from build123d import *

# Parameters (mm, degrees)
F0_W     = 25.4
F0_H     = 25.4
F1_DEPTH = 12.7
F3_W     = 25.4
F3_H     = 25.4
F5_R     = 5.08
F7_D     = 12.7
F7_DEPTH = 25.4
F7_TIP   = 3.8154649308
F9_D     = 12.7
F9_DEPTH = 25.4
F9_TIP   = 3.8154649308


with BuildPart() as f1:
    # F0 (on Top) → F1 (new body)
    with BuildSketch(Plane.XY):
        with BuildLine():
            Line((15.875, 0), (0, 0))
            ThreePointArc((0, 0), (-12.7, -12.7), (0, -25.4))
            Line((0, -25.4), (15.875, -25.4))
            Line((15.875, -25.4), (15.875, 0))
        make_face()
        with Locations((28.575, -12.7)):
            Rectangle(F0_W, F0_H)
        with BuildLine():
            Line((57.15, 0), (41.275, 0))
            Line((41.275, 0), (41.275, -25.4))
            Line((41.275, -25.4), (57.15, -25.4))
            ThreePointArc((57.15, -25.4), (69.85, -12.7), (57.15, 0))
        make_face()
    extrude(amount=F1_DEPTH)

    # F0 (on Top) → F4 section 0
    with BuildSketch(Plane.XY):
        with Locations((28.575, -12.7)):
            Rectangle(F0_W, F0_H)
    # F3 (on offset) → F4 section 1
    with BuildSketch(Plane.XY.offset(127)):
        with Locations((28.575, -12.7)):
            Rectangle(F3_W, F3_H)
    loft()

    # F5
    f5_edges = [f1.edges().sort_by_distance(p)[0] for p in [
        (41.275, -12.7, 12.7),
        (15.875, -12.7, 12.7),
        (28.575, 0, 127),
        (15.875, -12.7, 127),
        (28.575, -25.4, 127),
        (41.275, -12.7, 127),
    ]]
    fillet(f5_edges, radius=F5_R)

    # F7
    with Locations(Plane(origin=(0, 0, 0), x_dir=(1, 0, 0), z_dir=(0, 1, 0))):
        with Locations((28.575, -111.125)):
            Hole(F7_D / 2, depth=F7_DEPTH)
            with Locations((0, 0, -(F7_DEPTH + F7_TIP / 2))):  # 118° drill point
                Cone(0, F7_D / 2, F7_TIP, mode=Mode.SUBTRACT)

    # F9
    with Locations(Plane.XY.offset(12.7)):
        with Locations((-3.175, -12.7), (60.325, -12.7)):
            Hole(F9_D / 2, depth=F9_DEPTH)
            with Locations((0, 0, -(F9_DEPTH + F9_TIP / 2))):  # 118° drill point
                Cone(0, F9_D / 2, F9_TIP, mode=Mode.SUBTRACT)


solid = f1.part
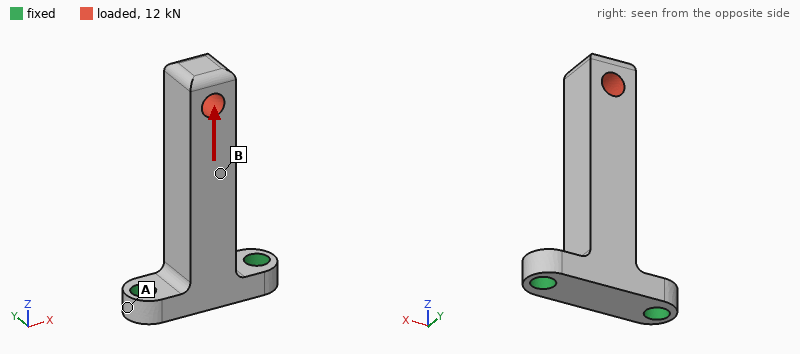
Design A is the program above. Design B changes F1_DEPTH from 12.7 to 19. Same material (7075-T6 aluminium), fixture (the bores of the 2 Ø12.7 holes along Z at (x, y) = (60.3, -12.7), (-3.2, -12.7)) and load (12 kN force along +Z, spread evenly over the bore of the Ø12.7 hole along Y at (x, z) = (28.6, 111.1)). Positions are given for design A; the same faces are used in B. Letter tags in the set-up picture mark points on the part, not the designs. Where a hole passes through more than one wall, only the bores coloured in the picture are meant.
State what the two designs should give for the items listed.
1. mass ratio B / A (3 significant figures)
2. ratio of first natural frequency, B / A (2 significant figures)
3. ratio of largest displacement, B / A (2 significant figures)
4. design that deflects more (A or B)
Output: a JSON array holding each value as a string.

["1.07", "1.3", "0.78", "A"]
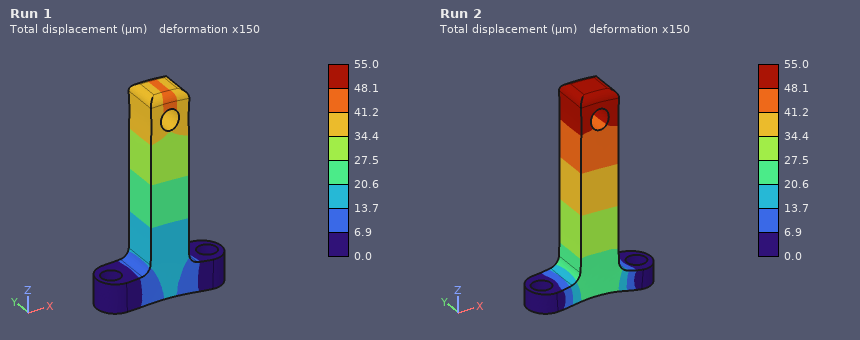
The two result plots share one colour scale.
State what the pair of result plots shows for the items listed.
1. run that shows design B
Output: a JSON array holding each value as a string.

["Run 1"]
